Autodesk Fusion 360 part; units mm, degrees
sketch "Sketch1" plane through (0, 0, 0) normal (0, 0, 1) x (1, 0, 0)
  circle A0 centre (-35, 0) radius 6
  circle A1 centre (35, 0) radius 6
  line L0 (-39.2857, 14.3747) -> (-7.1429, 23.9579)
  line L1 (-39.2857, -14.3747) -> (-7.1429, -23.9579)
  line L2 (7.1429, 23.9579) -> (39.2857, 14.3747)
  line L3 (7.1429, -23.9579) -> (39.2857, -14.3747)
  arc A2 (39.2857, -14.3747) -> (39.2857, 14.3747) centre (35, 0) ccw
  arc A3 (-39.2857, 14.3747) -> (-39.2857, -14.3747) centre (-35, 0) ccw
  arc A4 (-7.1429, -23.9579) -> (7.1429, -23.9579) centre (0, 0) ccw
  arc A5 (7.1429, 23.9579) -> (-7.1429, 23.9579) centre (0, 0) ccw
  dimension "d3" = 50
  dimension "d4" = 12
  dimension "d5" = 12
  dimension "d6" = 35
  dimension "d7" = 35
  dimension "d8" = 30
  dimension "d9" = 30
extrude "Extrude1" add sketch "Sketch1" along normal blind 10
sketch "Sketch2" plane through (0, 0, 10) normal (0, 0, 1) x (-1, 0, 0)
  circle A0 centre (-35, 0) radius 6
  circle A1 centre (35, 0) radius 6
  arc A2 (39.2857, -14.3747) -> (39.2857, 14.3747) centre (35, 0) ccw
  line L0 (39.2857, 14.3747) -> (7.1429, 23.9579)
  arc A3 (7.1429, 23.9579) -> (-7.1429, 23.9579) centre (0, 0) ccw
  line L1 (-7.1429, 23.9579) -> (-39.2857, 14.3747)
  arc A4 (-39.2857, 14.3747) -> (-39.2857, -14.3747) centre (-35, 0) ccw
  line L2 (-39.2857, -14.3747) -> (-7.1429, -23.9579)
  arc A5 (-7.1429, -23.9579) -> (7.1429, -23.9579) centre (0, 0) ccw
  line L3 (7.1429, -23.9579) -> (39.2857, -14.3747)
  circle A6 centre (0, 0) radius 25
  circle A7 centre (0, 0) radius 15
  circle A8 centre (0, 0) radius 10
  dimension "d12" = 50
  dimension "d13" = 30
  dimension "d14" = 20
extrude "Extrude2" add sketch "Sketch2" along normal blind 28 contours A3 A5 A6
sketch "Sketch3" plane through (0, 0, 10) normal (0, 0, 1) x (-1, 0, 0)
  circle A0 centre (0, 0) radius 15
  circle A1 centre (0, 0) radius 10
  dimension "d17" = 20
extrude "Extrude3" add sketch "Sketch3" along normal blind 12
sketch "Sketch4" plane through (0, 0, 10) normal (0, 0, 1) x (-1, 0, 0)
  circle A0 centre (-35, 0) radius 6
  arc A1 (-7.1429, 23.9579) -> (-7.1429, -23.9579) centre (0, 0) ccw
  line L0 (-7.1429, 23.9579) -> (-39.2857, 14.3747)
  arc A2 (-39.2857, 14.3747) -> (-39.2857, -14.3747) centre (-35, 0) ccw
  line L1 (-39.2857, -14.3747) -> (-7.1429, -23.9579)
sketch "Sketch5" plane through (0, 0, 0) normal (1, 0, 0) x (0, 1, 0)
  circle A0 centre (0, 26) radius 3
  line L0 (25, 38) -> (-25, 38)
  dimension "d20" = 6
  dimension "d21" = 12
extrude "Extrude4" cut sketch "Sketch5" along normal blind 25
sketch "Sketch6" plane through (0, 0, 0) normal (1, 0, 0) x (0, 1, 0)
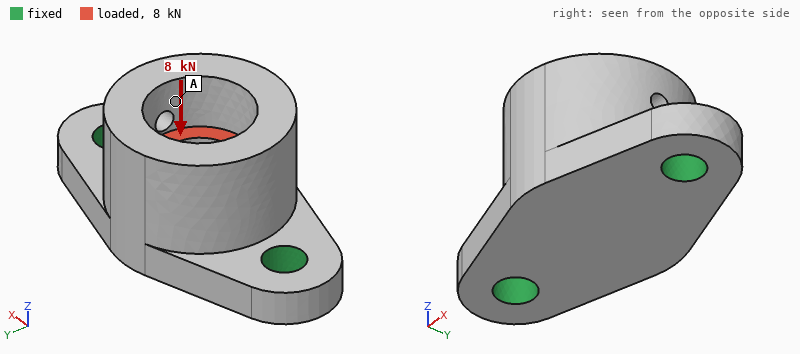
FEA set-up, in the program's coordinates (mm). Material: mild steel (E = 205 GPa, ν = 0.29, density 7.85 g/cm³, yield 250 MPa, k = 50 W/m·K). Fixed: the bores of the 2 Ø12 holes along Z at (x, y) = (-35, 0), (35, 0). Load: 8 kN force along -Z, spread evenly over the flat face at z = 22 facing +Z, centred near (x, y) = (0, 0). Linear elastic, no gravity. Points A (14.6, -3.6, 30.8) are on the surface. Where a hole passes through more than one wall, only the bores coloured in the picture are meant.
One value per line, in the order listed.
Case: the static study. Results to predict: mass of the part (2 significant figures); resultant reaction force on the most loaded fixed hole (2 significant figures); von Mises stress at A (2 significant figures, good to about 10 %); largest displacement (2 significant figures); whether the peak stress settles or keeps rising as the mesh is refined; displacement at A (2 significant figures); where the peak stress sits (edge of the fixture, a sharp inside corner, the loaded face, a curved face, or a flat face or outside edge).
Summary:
580 g
4.3 kN
9.9 MPa
5.9 µm
keeps rising
4.6 µm
edge of the fixture
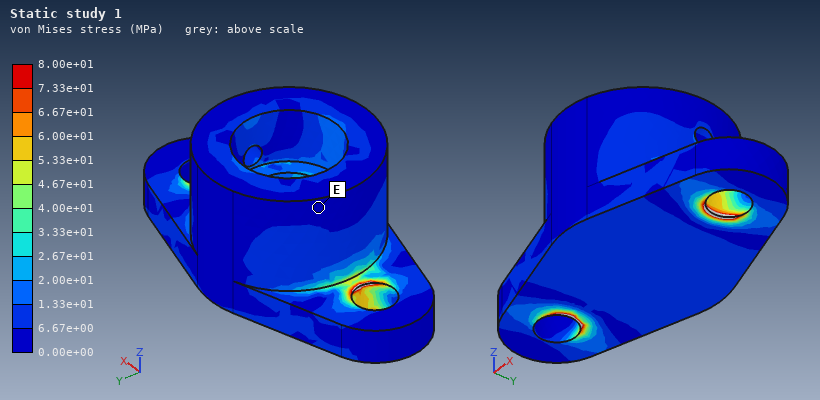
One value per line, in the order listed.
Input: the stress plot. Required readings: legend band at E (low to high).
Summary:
0.00e+00 to 6.67e+00 MPa
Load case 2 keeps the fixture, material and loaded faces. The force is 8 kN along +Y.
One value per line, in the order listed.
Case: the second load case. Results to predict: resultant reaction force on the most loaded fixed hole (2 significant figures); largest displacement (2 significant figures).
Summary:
4.0 kN
37 µm
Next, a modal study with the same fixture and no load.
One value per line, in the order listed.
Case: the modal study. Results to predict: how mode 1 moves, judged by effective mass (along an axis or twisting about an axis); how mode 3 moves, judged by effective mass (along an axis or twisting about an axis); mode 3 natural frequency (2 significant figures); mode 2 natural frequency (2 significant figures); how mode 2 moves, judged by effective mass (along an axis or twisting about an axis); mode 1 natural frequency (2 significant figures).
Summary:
along Y
along X
12 kHz
9300 Hz
along Z
4300 Hz
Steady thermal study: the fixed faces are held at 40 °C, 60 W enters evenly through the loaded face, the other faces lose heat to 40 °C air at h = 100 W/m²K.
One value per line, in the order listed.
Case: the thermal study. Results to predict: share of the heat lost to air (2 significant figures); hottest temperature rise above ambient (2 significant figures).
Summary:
39 %
35 K
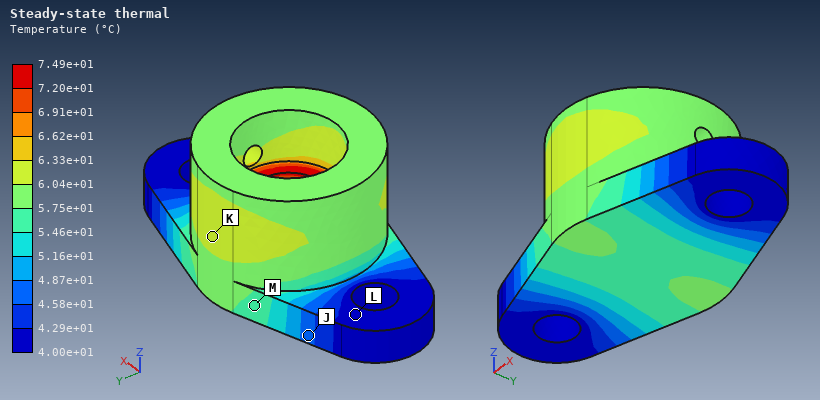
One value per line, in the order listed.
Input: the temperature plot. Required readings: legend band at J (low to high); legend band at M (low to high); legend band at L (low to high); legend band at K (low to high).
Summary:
4.58e+01 to 4.87e+01 °C
5.46e+01 to 5.75e+01 °C
4.00e+01 to 4.29e+01 °C
6.04e+01 to 6.33e+01 °C
